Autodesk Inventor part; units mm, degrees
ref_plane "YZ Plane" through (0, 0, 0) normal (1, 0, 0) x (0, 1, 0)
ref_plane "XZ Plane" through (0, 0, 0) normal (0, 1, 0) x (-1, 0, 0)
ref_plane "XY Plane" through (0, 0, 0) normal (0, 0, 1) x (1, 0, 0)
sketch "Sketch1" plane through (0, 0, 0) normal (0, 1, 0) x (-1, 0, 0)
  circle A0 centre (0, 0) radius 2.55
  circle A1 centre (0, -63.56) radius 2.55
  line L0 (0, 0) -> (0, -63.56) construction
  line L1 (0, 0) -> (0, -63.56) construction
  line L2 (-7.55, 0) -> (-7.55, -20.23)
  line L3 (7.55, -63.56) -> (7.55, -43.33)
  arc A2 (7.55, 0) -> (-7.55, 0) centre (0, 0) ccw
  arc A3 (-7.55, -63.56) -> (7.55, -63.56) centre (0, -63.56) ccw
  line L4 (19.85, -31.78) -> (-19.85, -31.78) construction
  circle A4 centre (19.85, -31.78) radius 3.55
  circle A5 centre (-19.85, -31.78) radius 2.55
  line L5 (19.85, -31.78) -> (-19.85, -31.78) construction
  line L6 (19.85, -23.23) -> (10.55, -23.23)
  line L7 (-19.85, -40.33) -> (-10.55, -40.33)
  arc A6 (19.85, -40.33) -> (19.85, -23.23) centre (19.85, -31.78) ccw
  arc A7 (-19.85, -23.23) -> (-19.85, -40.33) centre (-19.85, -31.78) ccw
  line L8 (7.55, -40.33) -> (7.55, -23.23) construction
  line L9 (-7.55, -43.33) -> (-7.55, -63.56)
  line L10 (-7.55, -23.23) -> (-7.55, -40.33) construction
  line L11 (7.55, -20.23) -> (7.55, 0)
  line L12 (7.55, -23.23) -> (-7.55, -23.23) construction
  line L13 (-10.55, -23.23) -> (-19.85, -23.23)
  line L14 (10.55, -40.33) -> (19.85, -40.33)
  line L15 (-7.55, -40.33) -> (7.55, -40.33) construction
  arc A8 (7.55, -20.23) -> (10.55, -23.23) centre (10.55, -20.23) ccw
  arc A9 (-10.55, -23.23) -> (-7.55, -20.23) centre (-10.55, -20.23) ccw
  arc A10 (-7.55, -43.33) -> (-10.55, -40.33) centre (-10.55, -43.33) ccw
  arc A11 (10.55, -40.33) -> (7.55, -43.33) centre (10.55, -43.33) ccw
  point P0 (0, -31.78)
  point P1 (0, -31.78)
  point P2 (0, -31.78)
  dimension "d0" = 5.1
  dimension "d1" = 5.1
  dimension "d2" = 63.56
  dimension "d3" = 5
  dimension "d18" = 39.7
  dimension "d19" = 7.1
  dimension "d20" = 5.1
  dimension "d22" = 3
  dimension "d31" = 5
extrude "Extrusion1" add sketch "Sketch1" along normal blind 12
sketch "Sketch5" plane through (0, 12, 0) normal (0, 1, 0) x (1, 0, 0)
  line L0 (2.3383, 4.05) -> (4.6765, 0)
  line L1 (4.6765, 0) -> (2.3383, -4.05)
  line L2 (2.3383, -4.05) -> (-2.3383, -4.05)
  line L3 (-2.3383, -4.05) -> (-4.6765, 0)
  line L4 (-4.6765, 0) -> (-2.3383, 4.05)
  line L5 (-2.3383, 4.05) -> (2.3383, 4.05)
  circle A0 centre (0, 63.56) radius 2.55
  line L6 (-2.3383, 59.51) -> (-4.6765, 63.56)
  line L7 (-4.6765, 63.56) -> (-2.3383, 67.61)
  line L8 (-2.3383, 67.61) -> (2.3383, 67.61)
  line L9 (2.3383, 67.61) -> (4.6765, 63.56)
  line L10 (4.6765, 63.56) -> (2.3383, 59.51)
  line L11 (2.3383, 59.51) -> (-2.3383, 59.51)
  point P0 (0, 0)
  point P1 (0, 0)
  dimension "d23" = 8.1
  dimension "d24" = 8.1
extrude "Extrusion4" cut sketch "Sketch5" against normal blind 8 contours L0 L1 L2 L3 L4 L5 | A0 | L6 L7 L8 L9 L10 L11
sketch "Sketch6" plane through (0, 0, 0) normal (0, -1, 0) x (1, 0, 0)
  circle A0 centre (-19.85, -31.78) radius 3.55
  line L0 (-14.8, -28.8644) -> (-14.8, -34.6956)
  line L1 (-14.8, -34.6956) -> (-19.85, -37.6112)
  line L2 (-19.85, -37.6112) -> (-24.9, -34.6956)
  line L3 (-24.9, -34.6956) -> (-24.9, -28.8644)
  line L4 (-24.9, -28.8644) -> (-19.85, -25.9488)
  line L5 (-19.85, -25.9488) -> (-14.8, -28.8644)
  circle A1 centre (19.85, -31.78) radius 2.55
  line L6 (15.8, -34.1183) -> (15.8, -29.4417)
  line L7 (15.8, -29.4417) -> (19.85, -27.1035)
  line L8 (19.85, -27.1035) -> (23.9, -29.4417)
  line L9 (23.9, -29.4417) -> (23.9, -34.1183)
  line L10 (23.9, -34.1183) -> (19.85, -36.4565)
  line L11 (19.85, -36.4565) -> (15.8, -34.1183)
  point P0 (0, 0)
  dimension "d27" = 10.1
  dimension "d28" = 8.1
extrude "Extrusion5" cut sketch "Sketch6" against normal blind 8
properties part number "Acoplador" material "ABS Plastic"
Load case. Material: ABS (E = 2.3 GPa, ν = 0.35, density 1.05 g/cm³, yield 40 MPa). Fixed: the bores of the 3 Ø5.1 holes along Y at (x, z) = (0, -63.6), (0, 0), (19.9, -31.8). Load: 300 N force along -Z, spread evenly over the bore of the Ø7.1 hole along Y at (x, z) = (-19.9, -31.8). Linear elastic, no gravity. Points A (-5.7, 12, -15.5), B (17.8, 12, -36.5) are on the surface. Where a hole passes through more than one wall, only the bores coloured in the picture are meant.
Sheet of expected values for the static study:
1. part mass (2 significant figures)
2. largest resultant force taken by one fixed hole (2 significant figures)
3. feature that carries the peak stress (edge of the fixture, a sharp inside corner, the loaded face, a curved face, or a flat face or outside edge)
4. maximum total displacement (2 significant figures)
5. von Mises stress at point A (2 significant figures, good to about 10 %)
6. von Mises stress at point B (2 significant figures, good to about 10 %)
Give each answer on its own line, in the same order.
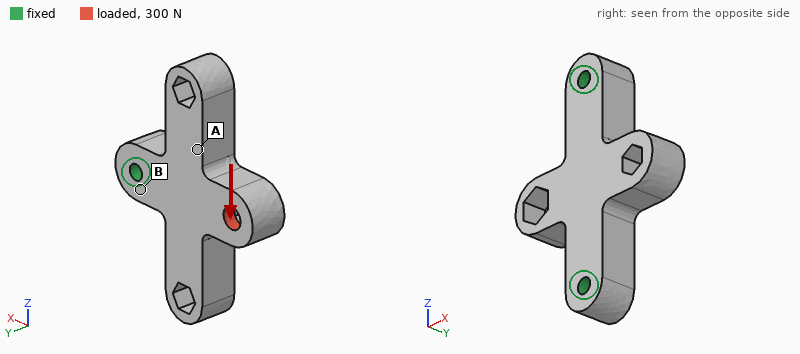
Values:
20 g
200 N
the loaded face
0.20 mm
2.6 MPa
1.5 MPa
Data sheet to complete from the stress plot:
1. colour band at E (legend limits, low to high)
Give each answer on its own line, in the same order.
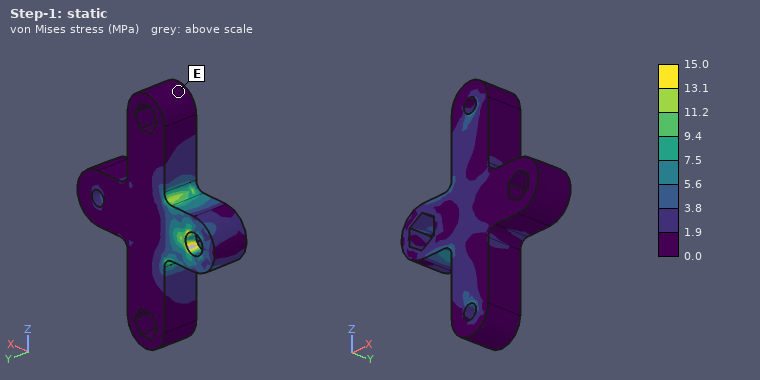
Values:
0.0 to 1.9 MPa
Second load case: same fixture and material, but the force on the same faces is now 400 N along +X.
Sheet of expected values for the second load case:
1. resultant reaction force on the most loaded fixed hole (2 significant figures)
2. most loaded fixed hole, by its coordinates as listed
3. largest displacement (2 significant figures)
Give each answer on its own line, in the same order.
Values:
340 N
(19.9, -31.8)
0.22 mm
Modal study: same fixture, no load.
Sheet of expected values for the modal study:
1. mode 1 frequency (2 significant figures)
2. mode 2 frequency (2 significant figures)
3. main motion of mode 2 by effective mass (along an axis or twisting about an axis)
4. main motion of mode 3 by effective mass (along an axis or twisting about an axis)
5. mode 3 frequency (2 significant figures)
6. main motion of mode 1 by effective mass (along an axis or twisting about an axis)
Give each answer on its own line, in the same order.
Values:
1900 Hz
4400 Hz
along Z
along X
5000 Hz
along Y
